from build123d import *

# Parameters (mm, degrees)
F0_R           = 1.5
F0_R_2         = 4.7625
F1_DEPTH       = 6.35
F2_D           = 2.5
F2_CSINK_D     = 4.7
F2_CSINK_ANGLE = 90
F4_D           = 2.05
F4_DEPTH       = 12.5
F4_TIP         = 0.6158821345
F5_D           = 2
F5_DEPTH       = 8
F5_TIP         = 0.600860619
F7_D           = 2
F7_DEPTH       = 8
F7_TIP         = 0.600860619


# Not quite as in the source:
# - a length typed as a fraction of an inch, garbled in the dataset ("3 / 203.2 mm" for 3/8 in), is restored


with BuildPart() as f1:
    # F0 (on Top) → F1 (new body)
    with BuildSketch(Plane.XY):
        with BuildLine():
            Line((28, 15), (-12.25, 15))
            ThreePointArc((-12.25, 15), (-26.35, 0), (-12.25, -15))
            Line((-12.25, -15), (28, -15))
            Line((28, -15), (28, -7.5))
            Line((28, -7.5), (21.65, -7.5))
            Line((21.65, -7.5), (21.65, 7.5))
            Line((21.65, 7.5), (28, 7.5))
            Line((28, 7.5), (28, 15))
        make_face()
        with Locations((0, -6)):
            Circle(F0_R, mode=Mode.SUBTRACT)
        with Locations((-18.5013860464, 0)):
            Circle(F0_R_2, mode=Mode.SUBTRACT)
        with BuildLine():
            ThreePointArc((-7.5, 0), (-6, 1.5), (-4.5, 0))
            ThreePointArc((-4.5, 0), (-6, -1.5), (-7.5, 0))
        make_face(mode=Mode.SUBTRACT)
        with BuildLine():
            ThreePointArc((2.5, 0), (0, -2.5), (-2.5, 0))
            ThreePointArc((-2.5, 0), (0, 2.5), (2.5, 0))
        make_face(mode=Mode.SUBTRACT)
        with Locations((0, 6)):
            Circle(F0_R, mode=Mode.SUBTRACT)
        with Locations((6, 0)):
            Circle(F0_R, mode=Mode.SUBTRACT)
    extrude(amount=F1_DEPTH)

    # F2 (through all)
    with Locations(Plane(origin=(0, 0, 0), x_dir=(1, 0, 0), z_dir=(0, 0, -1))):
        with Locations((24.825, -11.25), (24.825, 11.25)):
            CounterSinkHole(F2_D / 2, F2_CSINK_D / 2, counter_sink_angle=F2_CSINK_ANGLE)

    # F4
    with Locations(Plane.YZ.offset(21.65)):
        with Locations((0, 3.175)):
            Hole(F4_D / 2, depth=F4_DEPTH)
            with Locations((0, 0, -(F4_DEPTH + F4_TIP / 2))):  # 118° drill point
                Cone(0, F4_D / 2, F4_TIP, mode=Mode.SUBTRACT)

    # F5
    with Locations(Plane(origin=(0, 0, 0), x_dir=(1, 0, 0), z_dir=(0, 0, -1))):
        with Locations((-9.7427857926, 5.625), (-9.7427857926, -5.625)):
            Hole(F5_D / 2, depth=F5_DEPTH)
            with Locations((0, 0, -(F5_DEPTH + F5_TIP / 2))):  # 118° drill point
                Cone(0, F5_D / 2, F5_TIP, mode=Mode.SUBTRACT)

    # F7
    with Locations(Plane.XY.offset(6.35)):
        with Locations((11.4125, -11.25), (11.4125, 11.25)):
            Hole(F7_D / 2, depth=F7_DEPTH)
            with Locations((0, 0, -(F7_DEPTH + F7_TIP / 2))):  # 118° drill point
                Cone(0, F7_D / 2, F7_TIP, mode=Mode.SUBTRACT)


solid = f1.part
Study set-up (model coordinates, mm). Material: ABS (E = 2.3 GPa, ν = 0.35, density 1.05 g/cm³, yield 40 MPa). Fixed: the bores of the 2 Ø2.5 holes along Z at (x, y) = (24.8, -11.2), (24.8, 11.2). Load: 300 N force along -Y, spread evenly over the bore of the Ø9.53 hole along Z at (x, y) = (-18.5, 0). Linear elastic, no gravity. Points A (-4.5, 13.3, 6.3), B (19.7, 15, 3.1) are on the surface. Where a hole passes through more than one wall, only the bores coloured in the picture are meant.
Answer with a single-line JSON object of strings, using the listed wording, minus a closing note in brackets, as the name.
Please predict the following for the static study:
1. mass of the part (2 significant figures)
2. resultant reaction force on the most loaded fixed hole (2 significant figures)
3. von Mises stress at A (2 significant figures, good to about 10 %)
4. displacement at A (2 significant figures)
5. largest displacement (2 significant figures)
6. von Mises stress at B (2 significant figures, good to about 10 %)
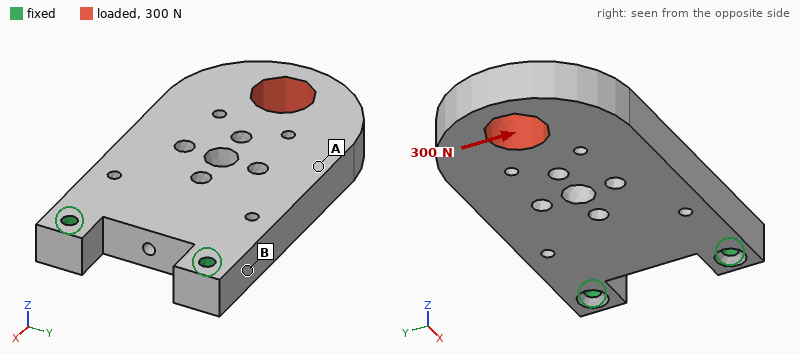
{"mass of the part": "8.6 g", "resultant reaction force on the most loaded fixed hole": "560 N", "von Mises stress at A": "3.7 MPa", "displacement at A": "0.29 mm", "largest displacement": "0.53 mm", "von Mises stress at B": "10.0 MPa"}
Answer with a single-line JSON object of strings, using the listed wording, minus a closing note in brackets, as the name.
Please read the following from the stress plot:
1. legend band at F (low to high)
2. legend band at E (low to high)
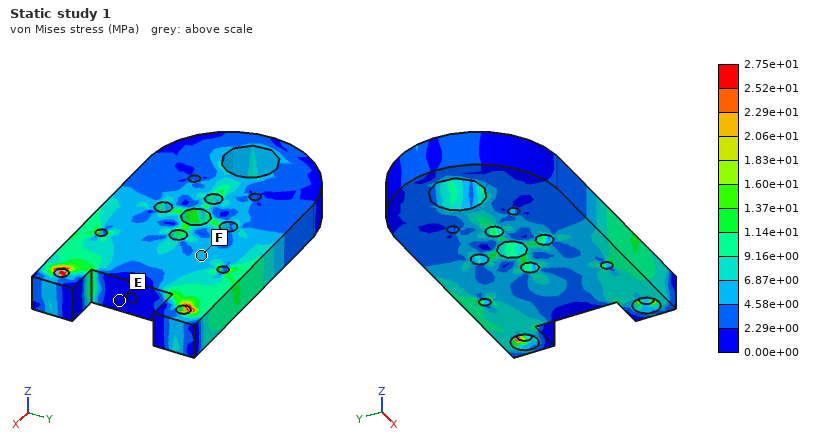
{"legend band at F": "4.58e+00 to 6.87e+00 MPa", "legend band at E": "0.00e+00 to 2.29e+00 MPa"}
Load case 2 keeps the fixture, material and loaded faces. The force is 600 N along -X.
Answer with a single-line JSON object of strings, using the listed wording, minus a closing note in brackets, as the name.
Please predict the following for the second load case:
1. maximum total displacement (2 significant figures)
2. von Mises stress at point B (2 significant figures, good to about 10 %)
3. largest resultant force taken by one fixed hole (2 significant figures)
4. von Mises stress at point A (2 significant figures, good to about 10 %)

{"maximum total displacement": "0.14 mm", "von Mises stress at point B": "4.2 MPa", "largest resultant force taken by one fixed hole": "310 N", "von Mises stress at point A": "3.3 MPa"}
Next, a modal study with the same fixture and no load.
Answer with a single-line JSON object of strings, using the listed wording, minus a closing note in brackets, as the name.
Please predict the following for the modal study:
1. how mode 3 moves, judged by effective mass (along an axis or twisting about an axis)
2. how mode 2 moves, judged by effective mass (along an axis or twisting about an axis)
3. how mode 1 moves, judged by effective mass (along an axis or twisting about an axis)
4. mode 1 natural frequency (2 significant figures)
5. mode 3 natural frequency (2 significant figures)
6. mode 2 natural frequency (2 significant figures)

{"how mode 3 moves, judged by effective mass": "along Y", "how mode 2 moves, judged by effective mass": "twisting about X", "how mode 1 moves, judged by effective mass": "along Z", "mode 1 natural frequency": "540 Hz", "mode 3 natural frequency": "2300 Hz", "mode 2 natural frequency": "2000 Hz"}
